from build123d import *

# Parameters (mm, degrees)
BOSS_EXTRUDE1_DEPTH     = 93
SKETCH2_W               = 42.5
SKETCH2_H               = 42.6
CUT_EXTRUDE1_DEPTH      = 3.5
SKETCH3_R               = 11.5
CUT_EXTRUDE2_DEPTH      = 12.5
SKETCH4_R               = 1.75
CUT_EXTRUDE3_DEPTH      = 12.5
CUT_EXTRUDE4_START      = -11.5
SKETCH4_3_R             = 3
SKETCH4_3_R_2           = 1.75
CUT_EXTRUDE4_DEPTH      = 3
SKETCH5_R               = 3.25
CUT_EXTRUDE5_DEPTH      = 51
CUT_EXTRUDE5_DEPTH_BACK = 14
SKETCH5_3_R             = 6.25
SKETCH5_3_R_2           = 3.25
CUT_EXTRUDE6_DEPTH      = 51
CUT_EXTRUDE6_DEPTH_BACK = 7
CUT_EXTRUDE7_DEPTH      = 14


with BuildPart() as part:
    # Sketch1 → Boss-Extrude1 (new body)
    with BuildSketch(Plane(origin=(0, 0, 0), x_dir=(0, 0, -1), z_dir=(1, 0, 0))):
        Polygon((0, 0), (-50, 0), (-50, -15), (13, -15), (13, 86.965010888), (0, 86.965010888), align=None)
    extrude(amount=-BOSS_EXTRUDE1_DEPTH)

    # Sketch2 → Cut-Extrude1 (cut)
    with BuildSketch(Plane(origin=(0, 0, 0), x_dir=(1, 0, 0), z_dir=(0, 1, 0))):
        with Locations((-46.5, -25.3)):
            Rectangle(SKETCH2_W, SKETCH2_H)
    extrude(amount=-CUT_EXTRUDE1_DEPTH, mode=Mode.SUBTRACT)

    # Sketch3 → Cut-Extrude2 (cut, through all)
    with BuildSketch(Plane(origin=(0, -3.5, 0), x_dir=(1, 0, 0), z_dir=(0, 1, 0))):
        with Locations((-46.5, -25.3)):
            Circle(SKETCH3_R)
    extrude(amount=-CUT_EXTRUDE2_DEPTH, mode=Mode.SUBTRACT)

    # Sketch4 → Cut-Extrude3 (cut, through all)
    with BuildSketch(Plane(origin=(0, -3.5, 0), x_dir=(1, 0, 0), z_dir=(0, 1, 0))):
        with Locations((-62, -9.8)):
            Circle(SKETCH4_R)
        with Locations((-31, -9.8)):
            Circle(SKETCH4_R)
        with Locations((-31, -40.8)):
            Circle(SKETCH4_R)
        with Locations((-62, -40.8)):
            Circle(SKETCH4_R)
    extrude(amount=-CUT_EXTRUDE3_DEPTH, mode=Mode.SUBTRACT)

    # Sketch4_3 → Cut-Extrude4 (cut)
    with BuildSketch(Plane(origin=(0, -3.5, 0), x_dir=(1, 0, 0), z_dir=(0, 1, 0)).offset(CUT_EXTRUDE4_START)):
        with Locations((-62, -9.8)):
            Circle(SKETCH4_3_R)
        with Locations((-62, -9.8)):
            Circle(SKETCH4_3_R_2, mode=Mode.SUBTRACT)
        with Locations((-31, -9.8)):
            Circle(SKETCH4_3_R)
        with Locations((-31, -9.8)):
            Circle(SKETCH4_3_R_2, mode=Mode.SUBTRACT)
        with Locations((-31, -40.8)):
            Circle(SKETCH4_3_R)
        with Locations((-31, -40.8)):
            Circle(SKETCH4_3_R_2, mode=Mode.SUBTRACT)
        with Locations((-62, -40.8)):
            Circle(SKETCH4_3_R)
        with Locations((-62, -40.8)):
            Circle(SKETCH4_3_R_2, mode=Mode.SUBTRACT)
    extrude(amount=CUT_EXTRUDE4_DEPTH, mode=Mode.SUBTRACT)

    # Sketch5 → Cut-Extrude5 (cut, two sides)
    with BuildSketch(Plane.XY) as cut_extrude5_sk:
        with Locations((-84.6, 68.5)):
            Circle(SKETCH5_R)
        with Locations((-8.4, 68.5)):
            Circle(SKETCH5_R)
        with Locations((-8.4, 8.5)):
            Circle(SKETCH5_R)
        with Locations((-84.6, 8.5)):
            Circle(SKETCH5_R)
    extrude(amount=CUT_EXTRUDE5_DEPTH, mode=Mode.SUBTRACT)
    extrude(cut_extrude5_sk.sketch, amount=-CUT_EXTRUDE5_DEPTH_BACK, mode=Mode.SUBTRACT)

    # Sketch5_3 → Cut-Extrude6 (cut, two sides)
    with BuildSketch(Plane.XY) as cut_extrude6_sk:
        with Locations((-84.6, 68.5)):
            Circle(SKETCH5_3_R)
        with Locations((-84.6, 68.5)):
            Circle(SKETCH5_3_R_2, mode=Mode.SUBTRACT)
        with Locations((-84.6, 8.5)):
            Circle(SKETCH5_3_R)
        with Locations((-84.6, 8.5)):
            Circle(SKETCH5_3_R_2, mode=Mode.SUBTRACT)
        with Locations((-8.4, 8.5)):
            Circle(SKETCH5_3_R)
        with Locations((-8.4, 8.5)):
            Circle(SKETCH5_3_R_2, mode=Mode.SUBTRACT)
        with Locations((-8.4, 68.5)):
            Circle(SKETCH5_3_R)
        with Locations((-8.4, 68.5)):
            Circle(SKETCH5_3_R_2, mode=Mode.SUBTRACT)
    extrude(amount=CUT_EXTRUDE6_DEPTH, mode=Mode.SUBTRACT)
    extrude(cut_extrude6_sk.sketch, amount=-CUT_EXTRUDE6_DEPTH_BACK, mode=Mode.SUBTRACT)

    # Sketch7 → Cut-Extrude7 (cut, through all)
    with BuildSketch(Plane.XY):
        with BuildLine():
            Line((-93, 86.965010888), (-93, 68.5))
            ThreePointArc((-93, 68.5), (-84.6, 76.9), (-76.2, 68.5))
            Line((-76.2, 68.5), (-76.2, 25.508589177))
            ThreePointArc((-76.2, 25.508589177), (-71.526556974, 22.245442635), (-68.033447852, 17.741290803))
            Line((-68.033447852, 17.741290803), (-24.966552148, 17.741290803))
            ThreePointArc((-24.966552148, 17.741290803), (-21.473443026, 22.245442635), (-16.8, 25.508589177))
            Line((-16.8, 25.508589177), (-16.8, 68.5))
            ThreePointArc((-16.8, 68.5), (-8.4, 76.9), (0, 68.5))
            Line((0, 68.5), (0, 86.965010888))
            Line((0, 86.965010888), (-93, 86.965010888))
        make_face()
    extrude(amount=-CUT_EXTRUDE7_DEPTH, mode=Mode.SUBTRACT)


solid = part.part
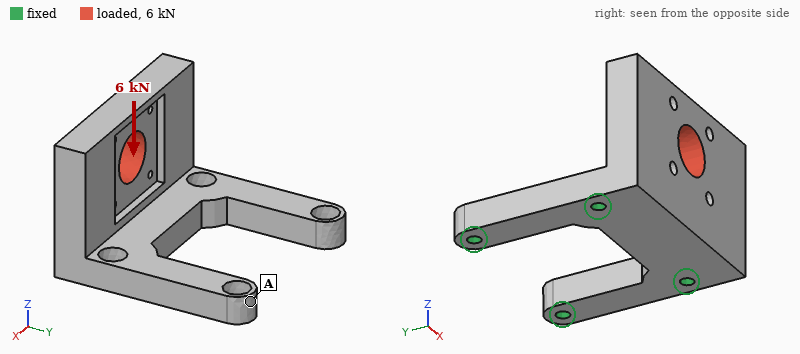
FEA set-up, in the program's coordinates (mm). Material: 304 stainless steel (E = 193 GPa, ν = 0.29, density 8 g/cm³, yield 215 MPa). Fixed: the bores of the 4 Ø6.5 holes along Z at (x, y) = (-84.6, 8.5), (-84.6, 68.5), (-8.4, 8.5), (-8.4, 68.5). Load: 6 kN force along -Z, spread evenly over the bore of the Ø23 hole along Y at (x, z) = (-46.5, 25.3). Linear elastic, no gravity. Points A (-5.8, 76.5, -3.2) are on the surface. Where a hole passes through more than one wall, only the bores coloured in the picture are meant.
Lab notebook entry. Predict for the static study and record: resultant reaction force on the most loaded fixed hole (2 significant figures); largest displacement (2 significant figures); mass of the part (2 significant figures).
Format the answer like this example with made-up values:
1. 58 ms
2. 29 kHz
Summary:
1. 3.7 kN
2. 72 µm
3. 950 g
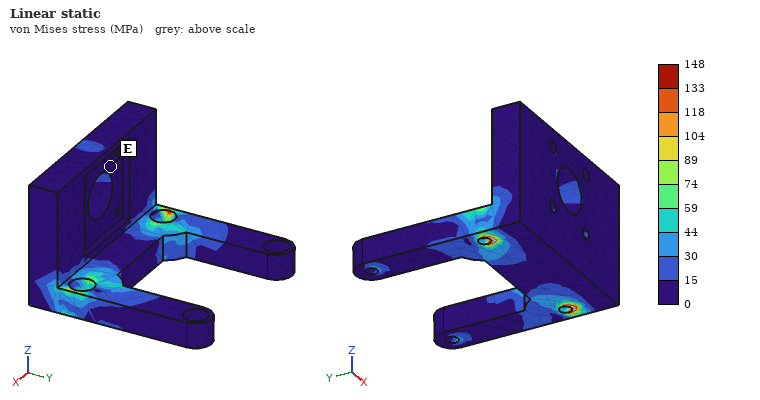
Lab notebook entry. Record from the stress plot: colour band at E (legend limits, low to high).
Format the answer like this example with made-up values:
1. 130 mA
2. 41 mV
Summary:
1. 0 to 15 MPa
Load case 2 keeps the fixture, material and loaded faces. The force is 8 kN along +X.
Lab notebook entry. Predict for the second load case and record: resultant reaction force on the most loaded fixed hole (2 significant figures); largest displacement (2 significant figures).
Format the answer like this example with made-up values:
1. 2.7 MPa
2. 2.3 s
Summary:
1. 5.7 kN
2. 27 µm
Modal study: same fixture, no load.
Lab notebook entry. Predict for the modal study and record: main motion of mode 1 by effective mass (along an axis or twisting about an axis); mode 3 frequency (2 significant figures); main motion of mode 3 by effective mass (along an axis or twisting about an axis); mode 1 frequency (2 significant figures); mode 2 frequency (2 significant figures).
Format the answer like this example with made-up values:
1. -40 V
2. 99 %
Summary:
1. along Y
2. 5800 Hz
3. along X
4. 1500 Hz
5. 3400 Hz
